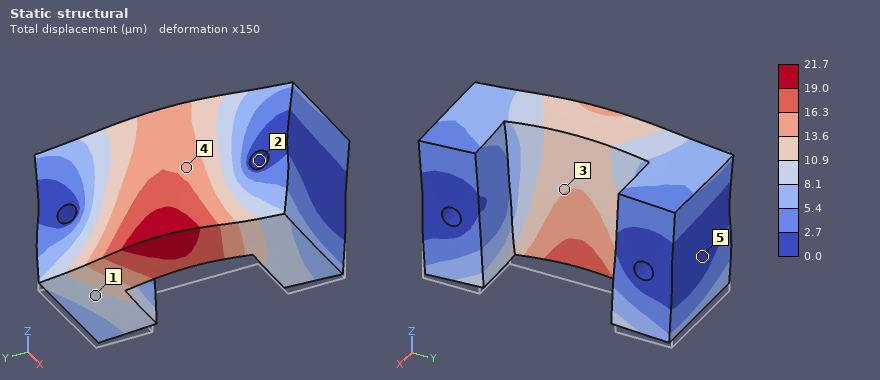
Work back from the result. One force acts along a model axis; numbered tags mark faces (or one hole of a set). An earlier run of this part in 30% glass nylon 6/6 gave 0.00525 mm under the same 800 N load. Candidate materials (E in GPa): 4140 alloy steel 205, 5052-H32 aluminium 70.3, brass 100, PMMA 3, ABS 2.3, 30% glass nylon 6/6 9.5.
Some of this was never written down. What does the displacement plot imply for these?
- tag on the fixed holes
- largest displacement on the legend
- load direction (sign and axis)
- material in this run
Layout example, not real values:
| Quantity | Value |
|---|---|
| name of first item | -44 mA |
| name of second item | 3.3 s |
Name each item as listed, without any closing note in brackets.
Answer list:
| Quantity | Value |
|---|---|
| tag on the fixed holes | 2 |
| largest displacement on the legend | 21.7 µm |
| load direction | +Z |
| material in this run | ABS |
